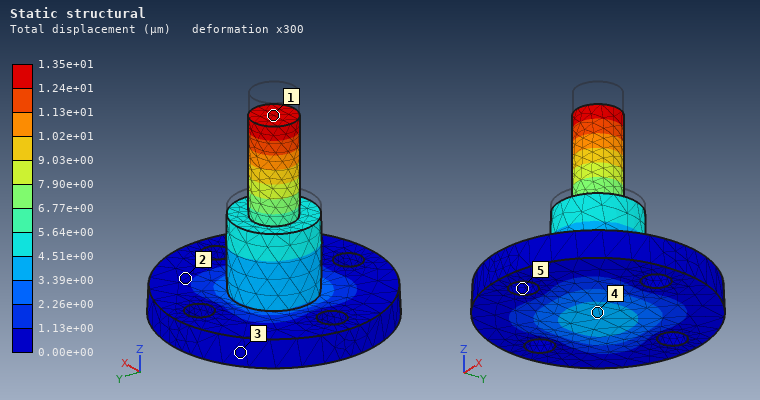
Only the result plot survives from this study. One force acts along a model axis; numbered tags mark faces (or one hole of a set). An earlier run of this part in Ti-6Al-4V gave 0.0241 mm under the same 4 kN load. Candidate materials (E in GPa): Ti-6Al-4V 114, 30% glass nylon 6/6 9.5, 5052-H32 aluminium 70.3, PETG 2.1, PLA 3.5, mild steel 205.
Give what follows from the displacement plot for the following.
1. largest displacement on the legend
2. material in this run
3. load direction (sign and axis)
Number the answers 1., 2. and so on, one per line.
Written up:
1. 1.35e+01 µm
2. mild steel
3. -Z
